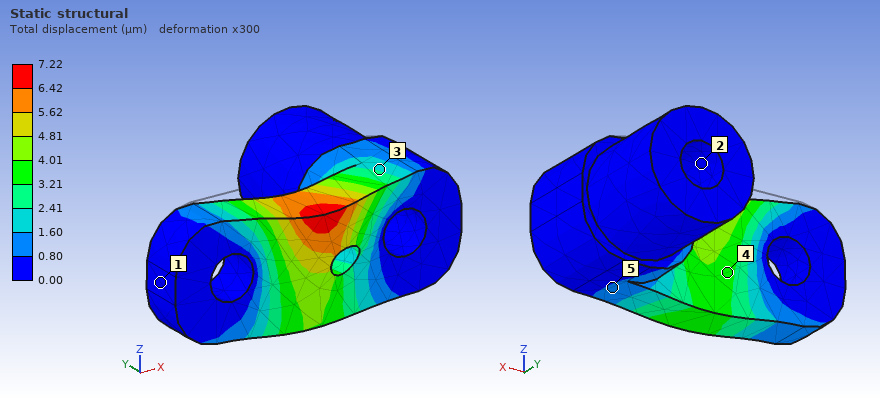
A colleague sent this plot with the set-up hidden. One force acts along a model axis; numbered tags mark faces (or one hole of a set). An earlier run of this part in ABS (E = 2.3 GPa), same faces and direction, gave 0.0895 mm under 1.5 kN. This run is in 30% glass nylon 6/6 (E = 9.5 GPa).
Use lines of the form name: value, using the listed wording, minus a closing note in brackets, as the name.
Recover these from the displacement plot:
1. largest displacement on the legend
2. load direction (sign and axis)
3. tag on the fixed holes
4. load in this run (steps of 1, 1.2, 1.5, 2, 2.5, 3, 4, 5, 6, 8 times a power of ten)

largest displacement on the legend: 7.22 µm
load direction: -Z
tag on the fixed holes: 2
load in this run: 500 N
